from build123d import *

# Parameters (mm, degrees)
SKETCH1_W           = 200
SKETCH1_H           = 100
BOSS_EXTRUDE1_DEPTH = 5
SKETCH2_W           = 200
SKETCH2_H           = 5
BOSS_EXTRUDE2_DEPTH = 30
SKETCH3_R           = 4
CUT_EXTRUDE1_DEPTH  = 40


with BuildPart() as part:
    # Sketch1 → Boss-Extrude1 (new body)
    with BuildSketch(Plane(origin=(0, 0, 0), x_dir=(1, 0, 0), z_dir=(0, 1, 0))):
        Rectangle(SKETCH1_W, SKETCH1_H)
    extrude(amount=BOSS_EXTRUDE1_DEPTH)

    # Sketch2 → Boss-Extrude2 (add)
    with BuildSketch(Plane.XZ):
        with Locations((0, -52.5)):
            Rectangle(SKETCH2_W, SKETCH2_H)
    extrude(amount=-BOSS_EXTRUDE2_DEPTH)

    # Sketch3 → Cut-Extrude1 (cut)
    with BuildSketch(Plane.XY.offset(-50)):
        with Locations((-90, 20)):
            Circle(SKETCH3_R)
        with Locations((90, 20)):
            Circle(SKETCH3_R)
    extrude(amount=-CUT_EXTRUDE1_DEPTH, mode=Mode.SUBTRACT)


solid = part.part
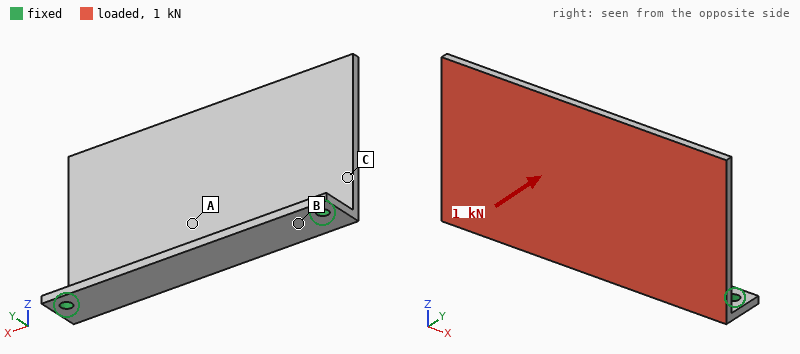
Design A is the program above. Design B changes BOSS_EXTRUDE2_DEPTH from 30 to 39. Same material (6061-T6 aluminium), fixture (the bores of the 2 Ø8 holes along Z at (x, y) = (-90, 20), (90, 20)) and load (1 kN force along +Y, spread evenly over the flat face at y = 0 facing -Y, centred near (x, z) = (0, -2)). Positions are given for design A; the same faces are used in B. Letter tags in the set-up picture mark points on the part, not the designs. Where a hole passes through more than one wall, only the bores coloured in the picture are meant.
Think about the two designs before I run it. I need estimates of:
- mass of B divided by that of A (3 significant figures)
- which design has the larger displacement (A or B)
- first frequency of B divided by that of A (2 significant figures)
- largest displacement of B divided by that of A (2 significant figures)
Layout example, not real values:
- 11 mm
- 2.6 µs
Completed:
- 1.07
- A
- 1.1
- 0.90
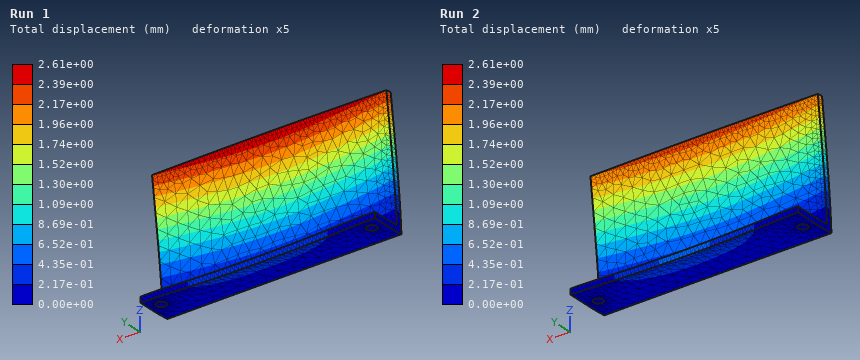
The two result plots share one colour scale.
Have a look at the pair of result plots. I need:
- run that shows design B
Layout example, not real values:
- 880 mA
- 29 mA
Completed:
- Run 2
